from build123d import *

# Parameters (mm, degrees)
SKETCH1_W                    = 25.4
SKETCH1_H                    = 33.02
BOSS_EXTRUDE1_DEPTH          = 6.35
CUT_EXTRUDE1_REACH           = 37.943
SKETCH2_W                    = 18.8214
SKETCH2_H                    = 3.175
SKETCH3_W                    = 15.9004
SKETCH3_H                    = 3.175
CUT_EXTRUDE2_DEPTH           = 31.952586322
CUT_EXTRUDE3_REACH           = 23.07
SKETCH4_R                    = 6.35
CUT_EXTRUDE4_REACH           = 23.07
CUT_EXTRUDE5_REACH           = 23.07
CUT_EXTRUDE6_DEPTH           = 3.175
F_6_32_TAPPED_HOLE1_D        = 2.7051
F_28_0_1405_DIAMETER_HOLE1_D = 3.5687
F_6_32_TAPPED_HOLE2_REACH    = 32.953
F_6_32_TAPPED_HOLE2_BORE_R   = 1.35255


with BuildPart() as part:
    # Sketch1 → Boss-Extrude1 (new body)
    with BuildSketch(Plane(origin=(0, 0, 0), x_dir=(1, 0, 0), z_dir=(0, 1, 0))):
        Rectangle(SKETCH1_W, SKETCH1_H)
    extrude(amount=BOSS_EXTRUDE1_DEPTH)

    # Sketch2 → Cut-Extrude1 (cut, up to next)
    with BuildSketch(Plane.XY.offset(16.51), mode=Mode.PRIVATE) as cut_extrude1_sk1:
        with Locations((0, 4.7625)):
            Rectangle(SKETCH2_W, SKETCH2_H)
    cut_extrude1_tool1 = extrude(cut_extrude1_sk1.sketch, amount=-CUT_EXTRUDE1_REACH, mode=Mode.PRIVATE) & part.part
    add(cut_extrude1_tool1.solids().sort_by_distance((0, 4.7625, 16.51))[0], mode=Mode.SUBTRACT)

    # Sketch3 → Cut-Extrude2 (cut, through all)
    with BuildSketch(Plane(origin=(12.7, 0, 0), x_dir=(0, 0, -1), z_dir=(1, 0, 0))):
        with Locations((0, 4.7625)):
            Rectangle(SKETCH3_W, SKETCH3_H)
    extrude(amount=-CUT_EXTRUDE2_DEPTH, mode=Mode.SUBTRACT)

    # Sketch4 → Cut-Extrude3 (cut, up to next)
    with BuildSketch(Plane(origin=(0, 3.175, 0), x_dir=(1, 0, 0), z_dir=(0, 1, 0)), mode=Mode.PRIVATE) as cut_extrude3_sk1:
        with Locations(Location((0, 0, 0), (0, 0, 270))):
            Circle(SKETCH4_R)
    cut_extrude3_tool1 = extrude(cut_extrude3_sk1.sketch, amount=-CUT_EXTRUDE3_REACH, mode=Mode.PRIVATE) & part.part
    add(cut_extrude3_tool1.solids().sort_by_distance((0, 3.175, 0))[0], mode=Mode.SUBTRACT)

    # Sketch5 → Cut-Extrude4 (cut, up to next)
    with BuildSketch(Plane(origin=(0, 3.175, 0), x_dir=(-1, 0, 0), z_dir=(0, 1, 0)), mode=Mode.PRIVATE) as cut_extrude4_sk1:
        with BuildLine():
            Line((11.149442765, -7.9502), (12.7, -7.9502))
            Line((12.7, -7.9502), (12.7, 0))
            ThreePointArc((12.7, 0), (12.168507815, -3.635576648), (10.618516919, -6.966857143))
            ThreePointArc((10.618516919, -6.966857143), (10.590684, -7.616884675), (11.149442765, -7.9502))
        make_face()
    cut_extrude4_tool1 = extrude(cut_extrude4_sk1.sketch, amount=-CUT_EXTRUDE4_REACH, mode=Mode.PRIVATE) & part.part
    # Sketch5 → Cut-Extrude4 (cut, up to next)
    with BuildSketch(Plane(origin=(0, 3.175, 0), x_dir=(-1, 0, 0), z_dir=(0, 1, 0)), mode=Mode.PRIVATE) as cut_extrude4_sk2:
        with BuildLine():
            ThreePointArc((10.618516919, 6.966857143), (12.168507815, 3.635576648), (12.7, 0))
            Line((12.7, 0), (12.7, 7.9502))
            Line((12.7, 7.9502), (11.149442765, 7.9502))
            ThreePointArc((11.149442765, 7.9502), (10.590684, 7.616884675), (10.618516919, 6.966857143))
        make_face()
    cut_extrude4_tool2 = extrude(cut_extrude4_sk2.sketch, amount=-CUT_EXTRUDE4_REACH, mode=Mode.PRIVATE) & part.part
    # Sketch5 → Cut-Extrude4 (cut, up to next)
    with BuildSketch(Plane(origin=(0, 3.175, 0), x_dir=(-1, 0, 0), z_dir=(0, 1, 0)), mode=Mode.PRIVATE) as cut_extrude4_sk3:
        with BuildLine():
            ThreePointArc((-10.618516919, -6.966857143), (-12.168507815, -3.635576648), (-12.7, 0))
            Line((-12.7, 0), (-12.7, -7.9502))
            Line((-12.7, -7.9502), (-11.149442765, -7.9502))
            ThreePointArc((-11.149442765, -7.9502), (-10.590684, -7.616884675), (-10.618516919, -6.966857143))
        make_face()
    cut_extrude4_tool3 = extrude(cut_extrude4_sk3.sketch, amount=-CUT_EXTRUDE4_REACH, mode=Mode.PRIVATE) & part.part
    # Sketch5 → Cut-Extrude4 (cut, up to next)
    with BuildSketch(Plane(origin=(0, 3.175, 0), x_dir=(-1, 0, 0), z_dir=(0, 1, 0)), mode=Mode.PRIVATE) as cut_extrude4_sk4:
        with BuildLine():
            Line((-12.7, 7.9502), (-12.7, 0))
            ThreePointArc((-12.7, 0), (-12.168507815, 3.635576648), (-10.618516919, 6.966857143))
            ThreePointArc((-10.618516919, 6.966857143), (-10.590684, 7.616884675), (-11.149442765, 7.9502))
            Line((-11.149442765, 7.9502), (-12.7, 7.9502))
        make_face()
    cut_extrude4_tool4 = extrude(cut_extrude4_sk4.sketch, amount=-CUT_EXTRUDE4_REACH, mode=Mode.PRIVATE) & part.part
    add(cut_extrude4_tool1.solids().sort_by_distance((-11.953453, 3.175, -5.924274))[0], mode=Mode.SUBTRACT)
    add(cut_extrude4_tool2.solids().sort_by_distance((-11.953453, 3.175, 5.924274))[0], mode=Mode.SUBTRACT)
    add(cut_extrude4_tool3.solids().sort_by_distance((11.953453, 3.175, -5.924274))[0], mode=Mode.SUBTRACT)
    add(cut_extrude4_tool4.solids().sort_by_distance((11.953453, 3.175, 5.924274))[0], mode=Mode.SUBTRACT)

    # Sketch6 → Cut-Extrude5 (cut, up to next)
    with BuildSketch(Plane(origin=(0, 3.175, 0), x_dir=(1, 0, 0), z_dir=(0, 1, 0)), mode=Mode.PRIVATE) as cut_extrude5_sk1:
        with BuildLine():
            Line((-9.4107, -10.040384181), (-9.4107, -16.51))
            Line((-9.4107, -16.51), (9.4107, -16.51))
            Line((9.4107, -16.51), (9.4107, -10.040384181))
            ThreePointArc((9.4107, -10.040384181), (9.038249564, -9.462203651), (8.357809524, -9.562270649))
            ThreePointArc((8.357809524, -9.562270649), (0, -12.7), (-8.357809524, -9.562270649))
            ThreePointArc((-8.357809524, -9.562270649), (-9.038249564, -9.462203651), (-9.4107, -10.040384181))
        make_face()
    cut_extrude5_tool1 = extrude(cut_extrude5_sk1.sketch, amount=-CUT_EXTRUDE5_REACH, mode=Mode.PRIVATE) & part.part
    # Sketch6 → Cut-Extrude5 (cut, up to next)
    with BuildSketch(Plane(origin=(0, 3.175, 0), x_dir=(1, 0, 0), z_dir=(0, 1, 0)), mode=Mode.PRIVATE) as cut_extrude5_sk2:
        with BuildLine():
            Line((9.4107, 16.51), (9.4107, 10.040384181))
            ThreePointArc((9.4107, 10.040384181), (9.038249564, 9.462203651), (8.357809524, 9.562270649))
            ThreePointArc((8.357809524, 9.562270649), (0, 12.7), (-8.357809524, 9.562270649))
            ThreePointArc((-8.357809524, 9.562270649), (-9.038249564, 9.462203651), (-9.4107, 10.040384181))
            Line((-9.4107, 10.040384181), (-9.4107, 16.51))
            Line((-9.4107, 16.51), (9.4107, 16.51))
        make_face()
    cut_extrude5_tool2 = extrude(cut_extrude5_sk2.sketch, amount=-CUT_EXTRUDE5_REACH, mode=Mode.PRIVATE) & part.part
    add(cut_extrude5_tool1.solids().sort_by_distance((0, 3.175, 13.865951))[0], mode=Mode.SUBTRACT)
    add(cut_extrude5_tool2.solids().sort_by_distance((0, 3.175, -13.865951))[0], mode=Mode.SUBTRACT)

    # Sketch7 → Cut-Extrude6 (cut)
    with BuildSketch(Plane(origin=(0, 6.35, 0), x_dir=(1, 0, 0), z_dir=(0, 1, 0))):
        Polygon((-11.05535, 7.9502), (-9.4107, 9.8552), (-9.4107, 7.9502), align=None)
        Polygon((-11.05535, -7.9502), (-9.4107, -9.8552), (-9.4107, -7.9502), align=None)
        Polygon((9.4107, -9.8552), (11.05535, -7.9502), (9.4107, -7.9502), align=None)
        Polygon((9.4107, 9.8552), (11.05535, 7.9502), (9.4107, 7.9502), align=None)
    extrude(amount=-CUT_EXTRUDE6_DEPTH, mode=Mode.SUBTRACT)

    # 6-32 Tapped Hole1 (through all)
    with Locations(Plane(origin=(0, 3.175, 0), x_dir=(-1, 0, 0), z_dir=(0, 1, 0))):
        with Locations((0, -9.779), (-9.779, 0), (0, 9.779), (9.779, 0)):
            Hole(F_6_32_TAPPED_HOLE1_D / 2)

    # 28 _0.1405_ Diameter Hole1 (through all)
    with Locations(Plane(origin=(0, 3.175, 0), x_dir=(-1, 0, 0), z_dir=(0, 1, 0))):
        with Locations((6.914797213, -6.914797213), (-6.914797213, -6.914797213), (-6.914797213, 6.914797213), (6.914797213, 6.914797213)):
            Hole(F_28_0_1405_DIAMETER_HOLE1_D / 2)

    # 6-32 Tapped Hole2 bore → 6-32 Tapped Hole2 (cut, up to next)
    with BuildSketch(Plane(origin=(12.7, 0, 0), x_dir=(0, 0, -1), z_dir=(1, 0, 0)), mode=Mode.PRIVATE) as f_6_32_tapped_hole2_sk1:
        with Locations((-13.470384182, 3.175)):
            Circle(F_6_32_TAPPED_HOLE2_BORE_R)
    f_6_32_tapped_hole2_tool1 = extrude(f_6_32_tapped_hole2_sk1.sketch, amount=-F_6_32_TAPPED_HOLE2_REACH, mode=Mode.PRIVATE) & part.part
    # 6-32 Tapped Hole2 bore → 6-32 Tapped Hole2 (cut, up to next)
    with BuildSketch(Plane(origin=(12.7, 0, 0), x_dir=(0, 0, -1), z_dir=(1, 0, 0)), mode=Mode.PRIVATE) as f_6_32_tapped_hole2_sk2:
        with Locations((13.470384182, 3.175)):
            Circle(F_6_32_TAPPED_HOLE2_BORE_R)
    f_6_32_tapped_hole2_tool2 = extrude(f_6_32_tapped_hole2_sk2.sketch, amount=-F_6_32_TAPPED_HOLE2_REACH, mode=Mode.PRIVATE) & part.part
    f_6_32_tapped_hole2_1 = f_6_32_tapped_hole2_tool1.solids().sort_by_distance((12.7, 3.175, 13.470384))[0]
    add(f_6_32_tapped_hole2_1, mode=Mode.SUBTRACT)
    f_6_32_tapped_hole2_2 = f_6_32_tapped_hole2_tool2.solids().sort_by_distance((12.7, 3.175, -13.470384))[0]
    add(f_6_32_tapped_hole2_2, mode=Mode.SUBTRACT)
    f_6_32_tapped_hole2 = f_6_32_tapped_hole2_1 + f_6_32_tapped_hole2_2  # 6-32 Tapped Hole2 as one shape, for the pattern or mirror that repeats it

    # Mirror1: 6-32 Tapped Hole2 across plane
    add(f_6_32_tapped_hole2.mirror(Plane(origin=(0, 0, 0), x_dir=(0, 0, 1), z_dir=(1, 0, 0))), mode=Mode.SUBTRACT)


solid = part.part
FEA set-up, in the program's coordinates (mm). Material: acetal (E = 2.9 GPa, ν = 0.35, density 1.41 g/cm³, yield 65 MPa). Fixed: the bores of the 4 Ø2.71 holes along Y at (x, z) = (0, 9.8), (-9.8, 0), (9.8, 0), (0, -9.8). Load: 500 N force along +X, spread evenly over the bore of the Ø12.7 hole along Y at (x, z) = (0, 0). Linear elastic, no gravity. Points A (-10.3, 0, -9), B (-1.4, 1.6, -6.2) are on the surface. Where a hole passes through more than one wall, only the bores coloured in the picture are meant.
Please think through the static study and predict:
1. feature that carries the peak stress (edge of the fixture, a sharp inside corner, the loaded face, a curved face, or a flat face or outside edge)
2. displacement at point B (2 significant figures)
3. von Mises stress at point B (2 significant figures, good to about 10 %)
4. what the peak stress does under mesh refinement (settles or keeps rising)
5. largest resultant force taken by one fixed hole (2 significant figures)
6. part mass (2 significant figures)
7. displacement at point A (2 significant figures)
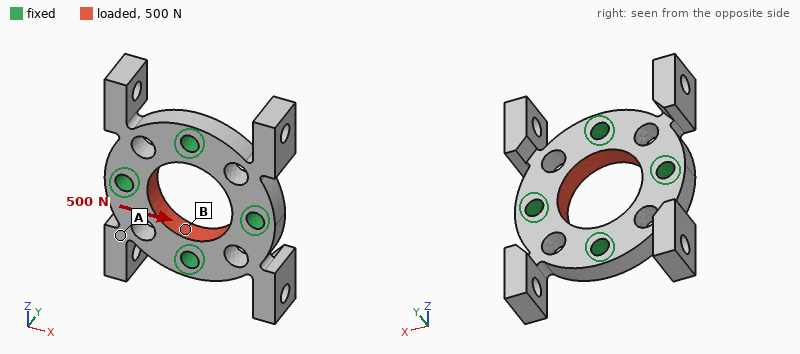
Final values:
edge of the fixture
15 µm
7.3 MPa
keeps rising
130 N
2.3 g
6.7 µm
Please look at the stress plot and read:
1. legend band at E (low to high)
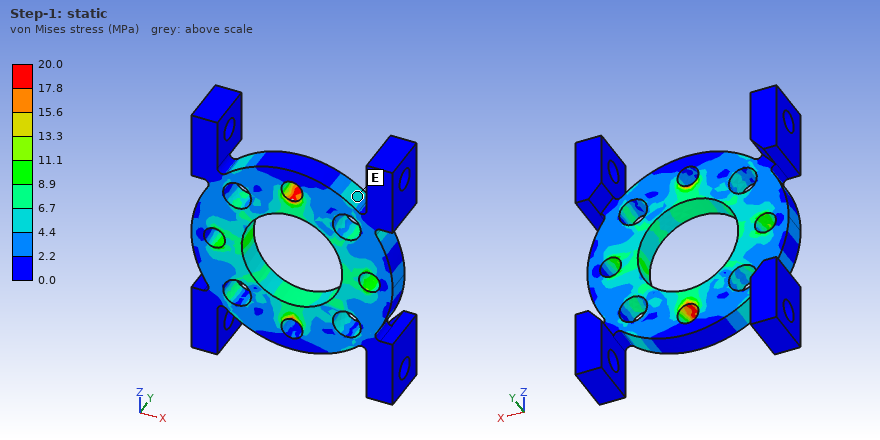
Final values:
4.4 to 6.7 MPa
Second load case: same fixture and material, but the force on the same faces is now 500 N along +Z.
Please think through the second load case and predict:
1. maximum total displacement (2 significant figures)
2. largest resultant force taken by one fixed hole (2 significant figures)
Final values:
21 µm
130 N
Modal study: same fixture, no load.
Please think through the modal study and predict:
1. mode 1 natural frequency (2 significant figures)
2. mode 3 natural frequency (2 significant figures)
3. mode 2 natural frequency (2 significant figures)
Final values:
2900 Hz
2900 Hz
2900 Hz
